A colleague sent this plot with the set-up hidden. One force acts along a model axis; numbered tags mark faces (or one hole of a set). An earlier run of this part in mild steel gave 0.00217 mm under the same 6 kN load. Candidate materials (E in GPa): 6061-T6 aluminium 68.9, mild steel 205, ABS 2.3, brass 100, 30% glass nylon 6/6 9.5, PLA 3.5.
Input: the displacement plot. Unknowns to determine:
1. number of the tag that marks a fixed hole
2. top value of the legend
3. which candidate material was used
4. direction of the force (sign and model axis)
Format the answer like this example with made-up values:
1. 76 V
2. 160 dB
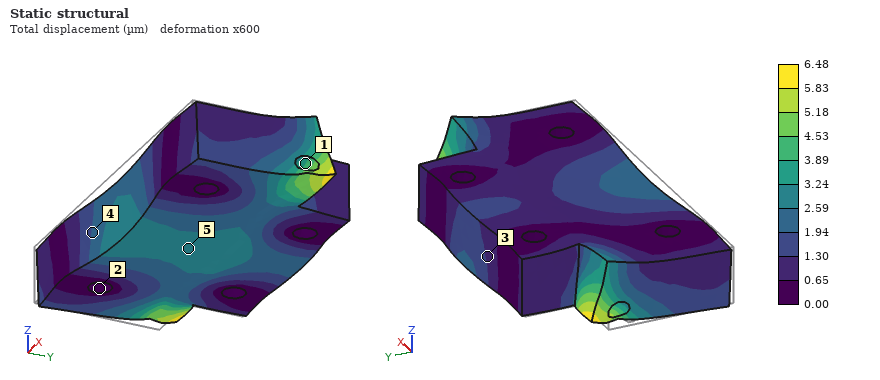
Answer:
1. 2
2. 6.48 µm
3. 6061-T6 aluminium
4. +Y
